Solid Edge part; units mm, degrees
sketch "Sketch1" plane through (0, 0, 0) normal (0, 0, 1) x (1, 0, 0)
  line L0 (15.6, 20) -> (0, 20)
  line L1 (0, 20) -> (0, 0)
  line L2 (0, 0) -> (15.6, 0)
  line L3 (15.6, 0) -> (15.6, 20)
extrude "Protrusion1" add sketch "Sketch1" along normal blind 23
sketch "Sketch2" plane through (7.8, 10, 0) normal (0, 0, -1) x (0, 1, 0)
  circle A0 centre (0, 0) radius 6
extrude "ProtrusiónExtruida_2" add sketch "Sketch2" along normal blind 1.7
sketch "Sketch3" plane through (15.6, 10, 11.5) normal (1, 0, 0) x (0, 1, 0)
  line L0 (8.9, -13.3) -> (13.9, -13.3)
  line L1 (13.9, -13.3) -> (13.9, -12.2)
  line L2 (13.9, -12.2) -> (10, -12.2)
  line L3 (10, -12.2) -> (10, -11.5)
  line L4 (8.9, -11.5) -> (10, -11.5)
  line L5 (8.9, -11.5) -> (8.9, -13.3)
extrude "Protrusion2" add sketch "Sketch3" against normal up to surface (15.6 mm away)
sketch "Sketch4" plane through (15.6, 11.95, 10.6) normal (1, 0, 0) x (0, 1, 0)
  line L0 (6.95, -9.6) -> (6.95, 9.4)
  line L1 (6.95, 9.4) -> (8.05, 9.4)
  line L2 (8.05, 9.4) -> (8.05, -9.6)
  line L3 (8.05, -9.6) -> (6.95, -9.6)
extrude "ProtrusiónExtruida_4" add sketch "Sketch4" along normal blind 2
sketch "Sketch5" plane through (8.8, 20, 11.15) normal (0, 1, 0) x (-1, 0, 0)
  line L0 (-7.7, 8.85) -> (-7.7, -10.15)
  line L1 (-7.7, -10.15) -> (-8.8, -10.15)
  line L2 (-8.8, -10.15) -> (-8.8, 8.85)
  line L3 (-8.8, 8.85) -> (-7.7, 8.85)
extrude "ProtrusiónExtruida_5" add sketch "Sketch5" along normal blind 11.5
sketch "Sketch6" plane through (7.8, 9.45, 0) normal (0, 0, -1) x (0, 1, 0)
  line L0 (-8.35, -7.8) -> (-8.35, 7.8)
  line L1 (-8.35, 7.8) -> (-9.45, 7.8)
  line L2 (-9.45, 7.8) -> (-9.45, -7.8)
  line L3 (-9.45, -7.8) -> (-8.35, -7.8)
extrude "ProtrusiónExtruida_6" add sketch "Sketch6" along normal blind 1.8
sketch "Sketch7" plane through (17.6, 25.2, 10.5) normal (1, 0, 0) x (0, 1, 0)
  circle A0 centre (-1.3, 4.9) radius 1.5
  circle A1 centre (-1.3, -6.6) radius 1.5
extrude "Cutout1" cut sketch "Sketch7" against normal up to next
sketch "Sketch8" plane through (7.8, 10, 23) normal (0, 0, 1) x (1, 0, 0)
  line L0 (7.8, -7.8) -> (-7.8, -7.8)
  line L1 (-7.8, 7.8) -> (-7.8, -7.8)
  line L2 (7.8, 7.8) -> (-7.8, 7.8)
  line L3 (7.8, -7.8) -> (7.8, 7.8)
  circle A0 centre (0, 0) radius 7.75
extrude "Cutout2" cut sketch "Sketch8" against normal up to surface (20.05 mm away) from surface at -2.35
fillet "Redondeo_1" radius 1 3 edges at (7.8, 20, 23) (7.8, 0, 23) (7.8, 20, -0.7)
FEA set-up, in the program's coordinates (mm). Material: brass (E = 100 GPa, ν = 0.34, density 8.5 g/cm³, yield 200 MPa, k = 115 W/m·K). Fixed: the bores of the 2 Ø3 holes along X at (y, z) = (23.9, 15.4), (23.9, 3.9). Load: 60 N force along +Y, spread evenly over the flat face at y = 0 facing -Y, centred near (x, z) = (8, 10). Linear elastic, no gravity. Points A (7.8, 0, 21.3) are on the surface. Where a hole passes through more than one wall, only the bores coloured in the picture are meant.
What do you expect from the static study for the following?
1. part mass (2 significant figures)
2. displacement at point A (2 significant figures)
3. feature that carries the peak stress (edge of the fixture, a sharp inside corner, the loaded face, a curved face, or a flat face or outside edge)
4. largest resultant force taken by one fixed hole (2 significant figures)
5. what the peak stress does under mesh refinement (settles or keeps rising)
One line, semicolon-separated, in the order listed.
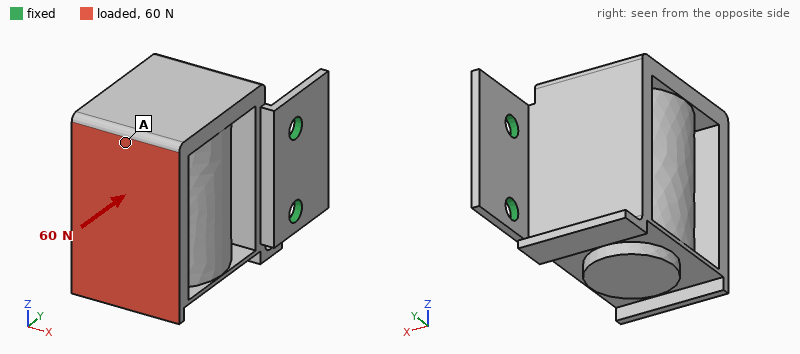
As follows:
57 g; 0.27 mm; edge of the fixture; 32 N; keeps rising
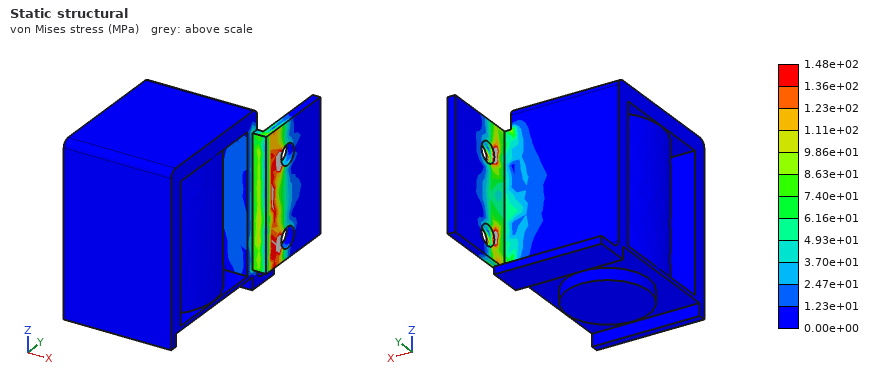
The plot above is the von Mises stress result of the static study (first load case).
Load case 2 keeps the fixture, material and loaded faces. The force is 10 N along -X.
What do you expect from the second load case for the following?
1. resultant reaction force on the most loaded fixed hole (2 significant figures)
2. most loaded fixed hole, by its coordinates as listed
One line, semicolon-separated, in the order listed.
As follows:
7.0 N; (23.9, 15.4)
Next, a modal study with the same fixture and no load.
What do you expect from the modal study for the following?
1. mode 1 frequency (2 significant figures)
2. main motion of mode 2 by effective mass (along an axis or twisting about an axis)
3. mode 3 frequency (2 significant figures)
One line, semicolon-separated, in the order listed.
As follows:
290 Hz; along Z; 2000 Hz
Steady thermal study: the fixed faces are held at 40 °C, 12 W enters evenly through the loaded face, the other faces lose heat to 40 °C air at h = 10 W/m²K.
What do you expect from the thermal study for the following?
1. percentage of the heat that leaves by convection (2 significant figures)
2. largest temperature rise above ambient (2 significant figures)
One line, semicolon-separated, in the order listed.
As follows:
13 %; 64 K
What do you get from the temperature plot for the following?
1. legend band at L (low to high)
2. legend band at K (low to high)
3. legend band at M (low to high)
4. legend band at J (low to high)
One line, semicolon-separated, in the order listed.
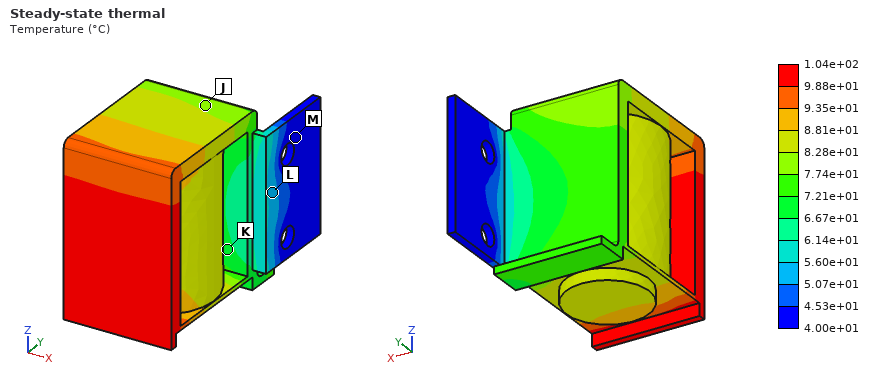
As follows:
5.07e+01 to 5.60e+01 °C; 6.67e+01 to 7.21e+01 °C; 4.00e+01 to 4.53e+01 °C; 7.74e+01 to 8.28e+01 °C
